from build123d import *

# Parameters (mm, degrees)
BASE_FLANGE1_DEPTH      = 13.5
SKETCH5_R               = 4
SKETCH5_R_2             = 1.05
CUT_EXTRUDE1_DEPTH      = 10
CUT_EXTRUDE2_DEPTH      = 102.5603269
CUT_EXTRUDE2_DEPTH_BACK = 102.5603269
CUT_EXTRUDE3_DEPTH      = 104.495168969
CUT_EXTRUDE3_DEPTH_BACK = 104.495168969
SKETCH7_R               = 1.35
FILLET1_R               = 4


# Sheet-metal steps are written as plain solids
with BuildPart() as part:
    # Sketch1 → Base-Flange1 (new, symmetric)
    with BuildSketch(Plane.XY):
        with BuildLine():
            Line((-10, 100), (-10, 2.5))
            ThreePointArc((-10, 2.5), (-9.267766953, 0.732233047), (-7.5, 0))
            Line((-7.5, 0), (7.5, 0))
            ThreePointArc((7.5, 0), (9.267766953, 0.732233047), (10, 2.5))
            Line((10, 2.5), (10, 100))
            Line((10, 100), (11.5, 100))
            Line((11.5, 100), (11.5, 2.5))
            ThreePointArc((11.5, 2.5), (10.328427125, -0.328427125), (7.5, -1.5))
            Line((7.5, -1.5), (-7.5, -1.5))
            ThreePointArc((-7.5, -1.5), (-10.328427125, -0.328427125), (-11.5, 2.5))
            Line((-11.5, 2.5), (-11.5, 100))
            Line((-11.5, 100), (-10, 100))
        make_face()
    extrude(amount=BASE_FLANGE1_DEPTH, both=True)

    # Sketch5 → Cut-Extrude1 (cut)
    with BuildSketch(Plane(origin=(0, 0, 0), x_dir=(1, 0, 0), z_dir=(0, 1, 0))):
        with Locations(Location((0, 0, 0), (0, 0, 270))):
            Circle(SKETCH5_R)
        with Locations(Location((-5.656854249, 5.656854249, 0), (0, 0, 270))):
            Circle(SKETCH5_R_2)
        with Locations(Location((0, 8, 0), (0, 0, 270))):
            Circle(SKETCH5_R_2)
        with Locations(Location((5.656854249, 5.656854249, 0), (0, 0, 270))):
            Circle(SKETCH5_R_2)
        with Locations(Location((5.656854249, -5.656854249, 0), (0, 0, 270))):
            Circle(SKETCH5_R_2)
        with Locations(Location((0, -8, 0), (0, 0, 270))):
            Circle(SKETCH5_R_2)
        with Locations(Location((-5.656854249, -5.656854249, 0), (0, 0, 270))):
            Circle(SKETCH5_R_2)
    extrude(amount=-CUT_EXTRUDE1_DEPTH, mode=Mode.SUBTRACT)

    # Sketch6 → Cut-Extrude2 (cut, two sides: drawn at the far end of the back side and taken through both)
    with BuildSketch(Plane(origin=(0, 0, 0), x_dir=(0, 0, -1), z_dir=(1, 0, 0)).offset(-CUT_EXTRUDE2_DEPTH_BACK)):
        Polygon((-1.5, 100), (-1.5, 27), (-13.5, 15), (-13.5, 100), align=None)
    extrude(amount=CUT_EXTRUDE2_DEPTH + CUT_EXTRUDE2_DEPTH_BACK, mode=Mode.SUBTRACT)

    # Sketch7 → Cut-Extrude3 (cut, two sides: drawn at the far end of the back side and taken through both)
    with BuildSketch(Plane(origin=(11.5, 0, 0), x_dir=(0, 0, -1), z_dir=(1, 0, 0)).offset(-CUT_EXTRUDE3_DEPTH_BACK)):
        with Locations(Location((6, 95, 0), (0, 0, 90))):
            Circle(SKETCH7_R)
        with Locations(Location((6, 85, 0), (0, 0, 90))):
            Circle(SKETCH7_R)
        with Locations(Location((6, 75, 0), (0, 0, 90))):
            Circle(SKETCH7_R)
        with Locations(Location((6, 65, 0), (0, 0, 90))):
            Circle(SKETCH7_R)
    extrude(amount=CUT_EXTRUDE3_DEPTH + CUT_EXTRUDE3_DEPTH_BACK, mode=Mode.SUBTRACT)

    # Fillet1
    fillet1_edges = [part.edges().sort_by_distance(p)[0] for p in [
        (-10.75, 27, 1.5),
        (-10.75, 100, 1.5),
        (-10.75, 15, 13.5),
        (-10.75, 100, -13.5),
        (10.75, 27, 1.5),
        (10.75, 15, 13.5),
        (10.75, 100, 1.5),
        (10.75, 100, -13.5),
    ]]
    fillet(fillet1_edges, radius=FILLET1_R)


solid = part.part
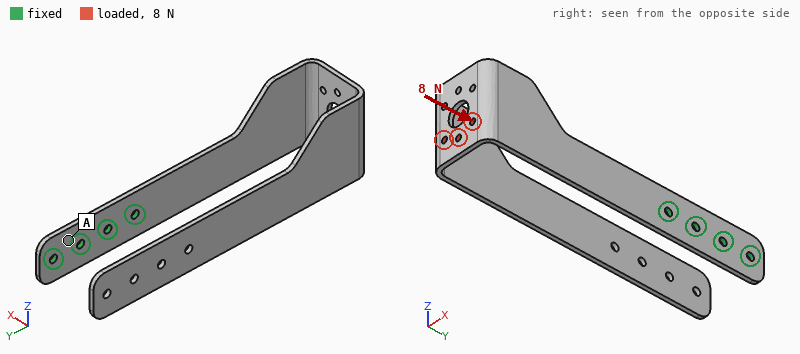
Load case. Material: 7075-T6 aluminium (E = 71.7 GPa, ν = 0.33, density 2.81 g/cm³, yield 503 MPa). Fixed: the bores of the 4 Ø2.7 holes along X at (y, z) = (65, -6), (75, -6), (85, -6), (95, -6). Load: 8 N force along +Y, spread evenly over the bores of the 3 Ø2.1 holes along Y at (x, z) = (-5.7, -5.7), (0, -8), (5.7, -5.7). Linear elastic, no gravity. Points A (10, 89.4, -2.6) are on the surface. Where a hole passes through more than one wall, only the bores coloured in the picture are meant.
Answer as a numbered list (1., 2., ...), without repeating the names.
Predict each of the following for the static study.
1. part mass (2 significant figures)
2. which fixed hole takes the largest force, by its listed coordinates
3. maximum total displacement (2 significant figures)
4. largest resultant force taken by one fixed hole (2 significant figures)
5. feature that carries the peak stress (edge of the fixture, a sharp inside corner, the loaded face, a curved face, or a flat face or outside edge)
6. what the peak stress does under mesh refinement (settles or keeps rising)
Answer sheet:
1. 17 g
2. (65, -6)
3. 1.2 mm
4. 6.5 N
5. edge of the fixture
6. keeps rising
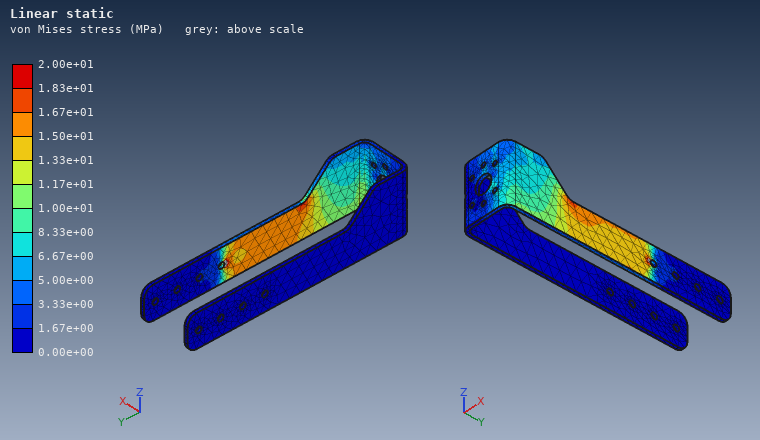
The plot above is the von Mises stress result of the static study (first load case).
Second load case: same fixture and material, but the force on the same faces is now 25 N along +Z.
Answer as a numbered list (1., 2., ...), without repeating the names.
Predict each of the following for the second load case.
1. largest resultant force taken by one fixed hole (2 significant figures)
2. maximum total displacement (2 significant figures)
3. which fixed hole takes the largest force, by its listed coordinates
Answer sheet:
1. 120 N
2. 1.1 mm
3. (65, -6)
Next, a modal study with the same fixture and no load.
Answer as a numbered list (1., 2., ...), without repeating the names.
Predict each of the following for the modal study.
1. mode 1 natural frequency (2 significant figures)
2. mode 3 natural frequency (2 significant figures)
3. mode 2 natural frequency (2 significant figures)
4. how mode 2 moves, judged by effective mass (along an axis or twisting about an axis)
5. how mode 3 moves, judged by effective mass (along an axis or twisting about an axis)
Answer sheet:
1. 80 Hz
2. 160 Hz
3. 130 Hz
4. along X
5. along Z
